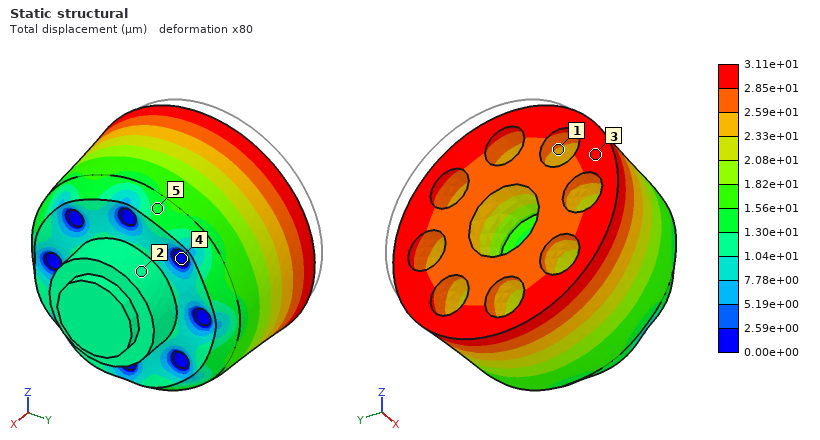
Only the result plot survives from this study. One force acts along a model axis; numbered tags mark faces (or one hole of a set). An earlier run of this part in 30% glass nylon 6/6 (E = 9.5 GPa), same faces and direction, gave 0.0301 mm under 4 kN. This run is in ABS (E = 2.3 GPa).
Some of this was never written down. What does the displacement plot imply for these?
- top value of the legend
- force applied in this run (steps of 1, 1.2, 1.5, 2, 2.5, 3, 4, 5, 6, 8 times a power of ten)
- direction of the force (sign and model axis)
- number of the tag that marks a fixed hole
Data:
3.11e+01 µm
1 kN
+X
4
